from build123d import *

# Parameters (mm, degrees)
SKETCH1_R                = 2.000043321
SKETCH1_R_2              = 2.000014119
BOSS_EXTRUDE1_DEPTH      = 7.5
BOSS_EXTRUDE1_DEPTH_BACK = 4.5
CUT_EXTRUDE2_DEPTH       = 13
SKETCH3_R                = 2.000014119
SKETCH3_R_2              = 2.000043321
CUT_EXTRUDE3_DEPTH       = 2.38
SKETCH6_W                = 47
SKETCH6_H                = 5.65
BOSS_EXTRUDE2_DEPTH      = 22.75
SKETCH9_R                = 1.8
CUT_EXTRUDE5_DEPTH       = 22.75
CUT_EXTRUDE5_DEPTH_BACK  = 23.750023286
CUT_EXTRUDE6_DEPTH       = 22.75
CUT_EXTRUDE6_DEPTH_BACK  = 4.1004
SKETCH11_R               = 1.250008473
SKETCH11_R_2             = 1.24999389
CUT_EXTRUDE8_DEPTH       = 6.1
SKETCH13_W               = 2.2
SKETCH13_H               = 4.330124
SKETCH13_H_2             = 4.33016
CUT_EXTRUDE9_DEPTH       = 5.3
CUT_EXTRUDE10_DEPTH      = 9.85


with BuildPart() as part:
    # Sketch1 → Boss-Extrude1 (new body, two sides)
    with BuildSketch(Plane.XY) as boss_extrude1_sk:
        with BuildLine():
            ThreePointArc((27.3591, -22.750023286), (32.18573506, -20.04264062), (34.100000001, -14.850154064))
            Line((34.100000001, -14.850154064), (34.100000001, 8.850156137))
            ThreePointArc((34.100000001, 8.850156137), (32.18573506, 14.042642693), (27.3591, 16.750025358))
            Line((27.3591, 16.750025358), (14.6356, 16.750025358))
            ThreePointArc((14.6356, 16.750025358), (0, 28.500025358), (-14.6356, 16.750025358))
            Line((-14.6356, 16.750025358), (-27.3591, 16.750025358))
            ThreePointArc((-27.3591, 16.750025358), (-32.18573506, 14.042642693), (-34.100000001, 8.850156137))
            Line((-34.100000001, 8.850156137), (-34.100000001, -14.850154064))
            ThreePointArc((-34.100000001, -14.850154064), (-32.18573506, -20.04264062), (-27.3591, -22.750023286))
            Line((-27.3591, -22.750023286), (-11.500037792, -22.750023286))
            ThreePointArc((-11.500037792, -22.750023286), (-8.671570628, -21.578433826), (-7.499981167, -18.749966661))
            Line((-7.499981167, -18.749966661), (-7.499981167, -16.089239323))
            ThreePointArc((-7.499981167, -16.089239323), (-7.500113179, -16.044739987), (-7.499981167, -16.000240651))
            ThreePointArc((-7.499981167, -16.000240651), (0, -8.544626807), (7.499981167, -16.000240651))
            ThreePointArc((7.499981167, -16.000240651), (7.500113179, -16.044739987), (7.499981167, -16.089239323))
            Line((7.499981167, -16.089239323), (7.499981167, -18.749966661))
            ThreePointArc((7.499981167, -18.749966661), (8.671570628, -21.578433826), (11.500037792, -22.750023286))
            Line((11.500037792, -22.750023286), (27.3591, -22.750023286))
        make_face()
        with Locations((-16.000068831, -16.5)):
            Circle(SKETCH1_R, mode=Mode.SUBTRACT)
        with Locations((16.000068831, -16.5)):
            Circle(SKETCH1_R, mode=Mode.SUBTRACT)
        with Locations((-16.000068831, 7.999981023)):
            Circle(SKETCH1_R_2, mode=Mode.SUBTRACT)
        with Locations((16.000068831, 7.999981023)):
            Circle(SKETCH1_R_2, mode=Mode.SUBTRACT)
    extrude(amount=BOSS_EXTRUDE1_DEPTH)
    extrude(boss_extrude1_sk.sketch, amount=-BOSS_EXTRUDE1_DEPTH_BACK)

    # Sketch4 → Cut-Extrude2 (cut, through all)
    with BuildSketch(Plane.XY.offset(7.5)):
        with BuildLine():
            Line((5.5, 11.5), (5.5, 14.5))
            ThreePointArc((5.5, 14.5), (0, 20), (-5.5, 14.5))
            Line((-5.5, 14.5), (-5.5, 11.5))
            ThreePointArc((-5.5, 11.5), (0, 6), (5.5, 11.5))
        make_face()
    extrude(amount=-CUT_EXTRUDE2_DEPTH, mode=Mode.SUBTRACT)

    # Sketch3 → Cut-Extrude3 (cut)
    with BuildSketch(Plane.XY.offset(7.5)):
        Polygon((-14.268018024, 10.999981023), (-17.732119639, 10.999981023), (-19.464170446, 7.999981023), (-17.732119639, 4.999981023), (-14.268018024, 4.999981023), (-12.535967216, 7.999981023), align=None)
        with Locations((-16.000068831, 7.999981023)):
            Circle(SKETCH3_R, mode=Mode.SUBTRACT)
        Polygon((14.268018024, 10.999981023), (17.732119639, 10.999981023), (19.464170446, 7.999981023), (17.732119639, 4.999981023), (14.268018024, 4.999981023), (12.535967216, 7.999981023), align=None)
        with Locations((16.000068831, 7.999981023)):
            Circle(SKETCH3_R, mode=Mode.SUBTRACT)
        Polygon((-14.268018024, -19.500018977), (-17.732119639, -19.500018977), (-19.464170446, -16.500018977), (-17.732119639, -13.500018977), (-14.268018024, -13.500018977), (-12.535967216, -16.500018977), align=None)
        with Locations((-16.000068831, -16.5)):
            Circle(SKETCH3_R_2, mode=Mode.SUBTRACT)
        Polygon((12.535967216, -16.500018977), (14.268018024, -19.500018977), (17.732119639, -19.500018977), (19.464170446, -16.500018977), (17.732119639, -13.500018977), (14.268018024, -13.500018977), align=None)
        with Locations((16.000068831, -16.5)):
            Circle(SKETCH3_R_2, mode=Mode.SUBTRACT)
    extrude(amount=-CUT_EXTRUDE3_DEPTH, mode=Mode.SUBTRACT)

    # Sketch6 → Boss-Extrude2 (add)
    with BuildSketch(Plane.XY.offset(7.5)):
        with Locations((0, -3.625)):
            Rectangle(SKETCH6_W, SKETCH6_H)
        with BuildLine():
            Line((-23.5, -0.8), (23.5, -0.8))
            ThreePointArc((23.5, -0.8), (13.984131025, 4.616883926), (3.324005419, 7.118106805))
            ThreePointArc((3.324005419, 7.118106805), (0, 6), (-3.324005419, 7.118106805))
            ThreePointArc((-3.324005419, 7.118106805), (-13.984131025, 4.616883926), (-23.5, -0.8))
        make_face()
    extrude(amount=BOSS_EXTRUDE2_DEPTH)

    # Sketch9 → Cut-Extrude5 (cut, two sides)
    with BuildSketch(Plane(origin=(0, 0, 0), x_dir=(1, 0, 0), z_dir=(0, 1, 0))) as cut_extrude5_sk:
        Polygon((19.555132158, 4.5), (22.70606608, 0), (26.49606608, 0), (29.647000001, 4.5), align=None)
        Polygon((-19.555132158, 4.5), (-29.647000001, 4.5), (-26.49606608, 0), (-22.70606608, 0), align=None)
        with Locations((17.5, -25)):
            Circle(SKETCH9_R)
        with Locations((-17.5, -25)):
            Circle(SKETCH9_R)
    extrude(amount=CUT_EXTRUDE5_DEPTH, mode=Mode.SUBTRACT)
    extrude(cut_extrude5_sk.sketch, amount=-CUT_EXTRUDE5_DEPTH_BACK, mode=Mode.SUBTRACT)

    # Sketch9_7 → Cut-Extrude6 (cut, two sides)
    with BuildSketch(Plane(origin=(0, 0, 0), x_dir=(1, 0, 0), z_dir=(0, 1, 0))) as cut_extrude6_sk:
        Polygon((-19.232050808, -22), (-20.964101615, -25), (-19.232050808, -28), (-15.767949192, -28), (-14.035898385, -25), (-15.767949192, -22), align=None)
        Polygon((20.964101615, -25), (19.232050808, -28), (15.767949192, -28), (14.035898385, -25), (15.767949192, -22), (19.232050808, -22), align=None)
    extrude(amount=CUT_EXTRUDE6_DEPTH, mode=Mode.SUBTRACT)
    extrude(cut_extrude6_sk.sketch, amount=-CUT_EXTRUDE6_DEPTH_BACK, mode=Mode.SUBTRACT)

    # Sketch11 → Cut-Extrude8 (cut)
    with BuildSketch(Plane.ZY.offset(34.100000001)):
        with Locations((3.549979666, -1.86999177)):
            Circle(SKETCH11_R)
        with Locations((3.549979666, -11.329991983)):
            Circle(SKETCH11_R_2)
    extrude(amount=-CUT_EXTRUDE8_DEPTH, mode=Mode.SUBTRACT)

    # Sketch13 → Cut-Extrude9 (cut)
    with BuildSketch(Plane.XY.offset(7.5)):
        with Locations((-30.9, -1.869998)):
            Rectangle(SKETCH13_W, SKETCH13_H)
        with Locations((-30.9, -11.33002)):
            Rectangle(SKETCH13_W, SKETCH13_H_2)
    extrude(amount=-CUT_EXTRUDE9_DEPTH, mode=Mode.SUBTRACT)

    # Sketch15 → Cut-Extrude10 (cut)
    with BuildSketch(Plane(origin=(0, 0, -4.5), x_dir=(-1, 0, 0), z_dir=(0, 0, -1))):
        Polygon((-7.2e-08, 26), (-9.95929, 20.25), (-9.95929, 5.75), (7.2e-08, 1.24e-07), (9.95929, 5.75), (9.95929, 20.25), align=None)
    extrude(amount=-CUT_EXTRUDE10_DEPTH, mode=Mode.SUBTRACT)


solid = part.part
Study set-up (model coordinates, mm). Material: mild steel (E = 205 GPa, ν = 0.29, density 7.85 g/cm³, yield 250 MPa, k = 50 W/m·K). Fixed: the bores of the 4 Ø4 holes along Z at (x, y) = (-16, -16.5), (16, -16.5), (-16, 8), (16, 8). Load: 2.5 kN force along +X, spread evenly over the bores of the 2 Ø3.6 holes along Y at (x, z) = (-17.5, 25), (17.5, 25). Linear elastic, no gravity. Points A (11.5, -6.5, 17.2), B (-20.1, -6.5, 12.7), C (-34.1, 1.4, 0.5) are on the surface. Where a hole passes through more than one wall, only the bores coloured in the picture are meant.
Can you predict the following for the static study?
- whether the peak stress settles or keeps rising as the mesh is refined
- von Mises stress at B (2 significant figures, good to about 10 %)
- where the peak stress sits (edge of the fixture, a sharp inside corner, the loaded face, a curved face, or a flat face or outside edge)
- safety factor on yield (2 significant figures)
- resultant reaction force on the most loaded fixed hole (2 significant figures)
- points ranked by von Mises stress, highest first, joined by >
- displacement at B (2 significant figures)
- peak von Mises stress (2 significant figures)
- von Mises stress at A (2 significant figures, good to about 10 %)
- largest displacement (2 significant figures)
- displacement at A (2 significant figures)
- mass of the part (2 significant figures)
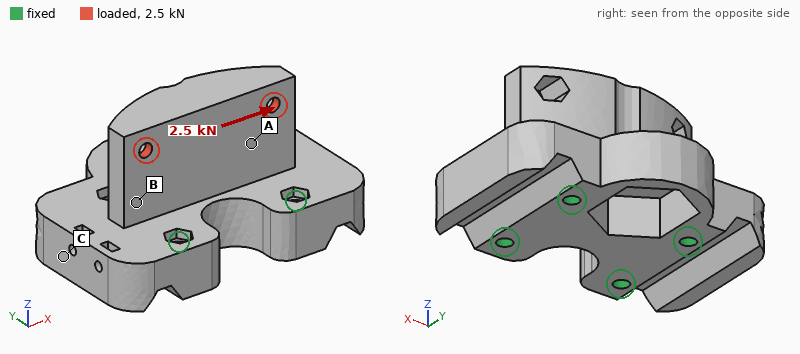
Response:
settles
12 MPa
the loaded face
2.5
1.4 kN
A > B > C
1.9 µm
100 MPa
22 MPa
6.9 µm
2.5 µm
280 g
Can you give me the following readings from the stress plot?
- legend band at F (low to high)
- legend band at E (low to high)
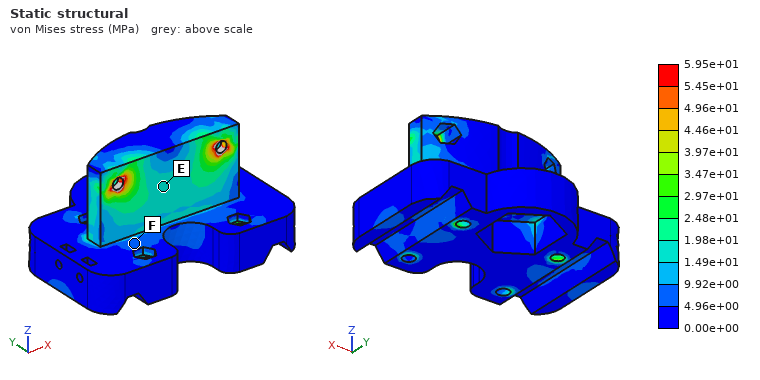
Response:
4.96e+00 to 9.92e+00 MPa
1.49e+01 to 1.98e+01 MPa
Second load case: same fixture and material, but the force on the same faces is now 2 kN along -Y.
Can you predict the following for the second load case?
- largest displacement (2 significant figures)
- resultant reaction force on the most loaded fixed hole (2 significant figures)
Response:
13 µm
1.1 kN
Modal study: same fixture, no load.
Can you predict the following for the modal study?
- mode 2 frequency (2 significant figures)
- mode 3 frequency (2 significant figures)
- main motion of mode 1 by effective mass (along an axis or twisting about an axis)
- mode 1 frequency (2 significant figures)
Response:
15 kHz
17 kHz
along Y
11 kHz
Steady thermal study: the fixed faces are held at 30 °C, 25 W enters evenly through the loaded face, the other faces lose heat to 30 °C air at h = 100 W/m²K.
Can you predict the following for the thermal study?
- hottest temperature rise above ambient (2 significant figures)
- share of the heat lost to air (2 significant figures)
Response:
47 K
30 %
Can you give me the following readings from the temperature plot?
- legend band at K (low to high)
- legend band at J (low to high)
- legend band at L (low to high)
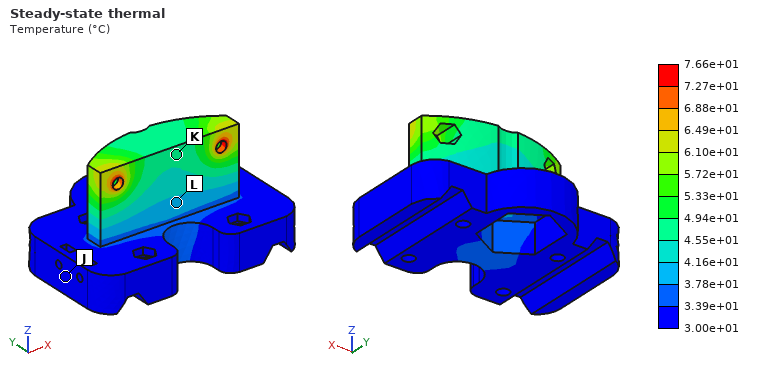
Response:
4.55e+01 to 4.94e+01 °C
3.00e+01 to 3.39e+01 °C
3.78e+01 to 4.16e+01 °C
